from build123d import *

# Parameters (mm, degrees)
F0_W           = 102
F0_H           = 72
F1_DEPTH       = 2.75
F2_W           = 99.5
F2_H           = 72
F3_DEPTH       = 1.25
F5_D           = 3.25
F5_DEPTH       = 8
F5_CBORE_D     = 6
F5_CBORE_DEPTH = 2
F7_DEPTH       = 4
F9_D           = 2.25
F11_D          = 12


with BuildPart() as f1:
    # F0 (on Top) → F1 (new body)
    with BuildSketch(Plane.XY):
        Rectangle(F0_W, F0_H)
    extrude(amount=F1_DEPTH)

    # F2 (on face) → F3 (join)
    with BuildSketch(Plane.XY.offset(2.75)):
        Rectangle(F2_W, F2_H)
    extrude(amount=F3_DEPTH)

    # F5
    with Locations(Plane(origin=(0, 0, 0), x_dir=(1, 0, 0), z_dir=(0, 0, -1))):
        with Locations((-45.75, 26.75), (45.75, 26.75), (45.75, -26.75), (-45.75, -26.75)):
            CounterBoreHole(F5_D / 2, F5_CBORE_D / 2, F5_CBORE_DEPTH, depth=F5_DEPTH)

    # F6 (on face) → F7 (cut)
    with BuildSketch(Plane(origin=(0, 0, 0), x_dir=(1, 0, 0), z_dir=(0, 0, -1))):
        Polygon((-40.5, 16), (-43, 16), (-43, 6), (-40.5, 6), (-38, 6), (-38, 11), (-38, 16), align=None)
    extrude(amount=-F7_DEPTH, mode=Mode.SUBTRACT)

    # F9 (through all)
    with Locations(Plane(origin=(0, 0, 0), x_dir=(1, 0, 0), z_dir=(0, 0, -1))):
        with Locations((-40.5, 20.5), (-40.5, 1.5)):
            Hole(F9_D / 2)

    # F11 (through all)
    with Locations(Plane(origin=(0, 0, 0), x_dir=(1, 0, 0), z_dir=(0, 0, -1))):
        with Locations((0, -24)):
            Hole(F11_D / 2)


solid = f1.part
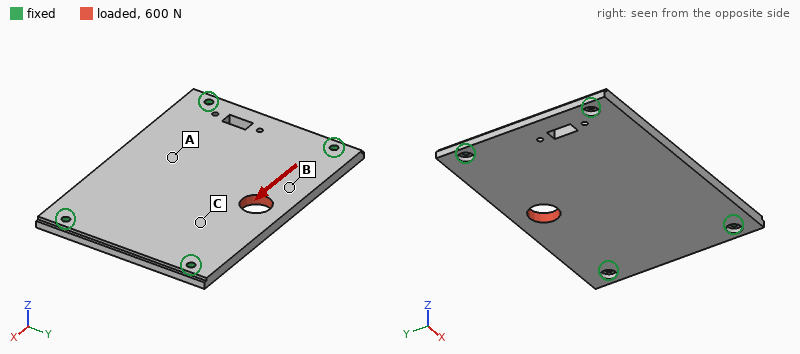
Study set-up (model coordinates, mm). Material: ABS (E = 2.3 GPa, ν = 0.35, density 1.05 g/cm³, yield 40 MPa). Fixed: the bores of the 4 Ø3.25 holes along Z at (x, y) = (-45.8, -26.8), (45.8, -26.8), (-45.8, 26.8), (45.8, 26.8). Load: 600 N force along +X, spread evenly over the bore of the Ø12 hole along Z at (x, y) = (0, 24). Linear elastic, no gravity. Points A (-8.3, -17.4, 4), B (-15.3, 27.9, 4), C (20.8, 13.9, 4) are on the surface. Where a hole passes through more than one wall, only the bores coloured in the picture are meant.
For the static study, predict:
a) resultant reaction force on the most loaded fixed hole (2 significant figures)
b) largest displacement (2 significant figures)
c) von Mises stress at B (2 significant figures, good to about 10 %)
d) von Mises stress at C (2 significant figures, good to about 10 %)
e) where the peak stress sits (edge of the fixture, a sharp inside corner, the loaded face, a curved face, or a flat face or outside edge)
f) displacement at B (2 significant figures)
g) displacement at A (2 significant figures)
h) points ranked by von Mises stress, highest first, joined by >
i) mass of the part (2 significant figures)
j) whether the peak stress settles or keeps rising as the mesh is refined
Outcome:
220 N
85 µm
3.7 MPa
2.0 MPa
edge of the fixture
67 µm
23 µm
B > C > A
30 g
keeps rising
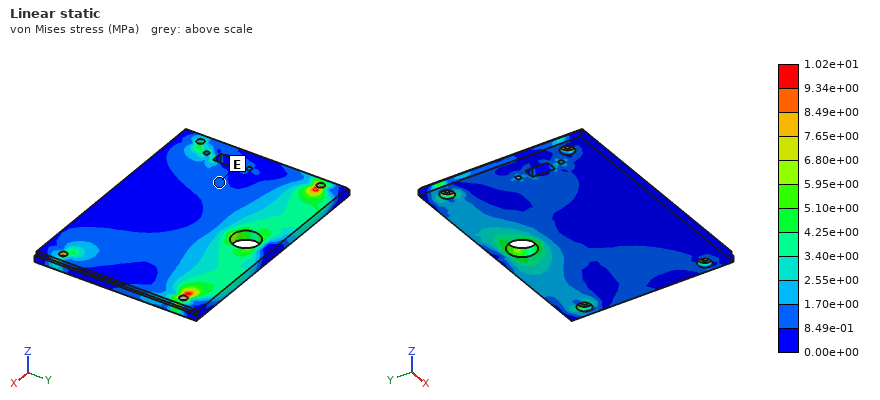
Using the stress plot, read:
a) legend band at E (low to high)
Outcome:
8.49e-01 to 1.70e+00 MPa
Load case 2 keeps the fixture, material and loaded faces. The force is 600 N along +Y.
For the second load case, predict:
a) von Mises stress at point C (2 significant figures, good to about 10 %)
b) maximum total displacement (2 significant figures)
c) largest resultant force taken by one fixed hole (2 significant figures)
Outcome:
3.0 MPa
0.16 mm
190 N
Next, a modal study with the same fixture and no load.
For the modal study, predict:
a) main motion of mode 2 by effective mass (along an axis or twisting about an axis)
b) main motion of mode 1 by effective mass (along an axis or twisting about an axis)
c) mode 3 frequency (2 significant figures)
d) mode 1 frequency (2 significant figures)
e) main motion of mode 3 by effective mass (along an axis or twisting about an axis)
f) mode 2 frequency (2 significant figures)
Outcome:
twisting about X
along Z
1400 Hz
510 Hz
twisting about Y
800 Hz
